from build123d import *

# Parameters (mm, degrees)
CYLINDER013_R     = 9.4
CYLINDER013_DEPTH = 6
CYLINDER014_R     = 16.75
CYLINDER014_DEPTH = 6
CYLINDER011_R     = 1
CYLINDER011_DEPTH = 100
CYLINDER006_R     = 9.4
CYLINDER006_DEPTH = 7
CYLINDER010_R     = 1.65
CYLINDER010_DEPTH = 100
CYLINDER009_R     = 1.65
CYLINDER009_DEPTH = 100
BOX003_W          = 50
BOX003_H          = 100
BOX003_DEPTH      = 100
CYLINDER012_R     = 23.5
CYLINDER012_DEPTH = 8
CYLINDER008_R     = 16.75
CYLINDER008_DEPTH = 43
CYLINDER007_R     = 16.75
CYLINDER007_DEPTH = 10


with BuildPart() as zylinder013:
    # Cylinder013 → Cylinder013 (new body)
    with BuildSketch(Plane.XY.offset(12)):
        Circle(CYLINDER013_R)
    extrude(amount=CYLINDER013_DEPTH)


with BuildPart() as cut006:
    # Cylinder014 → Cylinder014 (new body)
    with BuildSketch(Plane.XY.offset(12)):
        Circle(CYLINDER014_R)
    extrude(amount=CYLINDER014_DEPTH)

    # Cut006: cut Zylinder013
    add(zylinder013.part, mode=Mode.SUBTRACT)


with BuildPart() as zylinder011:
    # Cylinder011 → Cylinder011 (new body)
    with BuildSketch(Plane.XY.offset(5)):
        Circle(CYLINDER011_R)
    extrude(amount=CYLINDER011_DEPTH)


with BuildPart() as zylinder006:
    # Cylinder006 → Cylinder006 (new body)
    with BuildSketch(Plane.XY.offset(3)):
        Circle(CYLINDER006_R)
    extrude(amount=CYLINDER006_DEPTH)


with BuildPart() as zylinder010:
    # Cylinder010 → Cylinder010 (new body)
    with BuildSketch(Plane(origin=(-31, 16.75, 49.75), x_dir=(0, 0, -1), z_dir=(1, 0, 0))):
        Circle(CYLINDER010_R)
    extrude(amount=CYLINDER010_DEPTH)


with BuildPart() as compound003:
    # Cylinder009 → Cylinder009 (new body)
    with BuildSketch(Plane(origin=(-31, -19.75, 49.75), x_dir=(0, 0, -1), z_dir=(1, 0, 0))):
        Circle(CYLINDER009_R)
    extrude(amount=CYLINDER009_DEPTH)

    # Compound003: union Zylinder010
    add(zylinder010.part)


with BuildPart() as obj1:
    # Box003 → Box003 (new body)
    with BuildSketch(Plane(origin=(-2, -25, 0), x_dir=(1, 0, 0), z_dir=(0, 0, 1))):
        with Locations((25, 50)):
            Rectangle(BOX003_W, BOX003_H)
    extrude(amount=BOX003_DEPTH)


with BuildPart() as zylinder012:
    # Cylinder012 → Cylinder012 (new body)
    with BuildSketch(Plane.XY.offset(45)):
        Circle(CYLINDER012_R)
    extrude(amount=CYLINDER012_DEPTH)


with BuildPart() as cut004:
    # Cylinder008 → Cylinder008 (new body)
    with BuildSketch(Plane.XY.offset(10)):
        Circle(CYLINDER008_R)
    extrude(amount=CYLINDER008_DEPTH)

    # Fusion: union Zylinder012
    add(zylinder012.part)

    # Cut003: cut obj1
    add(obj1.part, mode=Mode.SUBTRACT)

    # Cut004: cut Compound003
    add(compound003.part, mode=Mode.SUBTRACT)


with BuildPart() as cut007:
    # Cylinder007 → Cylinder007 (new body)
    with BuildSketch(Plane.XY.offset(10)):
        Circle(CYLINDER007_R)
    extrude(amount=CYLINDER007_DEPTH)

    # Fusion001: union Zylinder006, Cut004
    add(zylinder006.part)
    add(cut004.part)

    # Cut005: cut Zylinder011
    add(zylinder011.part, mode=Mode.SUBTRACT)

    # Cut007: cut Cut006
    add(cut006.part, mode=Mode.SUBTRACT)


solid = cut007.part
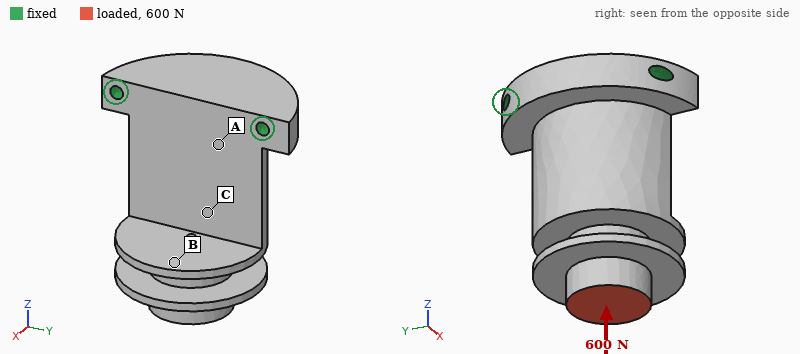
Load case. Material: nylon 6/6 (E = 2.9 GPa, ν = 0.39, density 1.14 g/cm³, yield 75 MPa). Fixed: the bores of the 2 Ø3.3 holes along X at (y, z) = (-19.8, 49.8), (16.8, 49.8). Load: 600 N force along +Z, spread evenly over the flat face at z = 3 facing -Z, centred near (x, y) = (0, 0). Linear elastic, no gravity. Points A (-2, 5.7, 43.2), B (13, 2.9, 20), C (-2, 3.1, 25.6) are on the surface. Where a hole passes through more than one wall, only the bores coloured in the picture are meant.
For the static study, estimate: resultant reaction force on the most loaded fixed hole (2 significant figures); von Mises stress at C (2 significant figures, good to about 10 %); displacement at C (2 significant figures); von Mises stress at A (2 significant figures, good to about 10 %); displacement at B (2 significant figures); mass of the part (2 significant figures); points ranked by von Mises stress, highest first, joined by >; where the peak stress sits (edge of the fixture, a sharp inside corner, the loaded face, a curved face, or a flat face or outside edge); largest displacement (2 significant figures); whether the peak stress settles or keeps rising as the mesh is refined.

350 N
9.8 MPa
0.23 mm
5.5 MPa
0.57 mm
26 g
C > A > B
edge of the fixture
0.78 mm
keeps rising
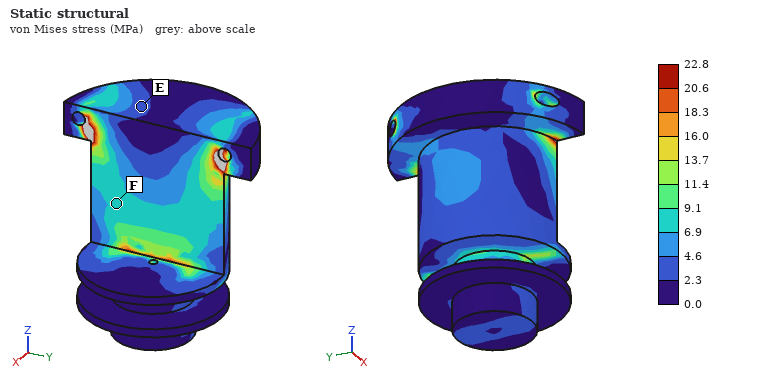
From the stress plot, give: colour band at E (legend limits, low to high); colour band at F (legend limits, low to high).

2.3 to 4.6 MPa
6.9 to 9.1 MPa
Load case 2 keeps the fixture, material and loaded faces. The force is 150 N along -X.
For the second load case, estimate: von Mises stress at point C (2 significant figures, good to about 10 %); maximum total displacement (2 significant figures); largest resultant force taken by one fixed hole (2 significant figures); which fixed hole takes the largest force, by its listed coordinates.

5.3 MPa
0.87 mm
100 N
(16.8, 49.8)
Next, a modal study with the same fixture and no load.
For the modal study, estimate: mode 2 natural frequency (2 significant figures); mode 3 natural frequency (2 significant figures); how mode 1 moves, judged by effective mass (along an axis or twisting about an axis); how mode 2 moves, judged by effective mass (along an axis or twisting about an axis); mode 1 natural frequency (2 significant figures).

2100 Hz
3000 Hz
along X
along Y
910 Hz
